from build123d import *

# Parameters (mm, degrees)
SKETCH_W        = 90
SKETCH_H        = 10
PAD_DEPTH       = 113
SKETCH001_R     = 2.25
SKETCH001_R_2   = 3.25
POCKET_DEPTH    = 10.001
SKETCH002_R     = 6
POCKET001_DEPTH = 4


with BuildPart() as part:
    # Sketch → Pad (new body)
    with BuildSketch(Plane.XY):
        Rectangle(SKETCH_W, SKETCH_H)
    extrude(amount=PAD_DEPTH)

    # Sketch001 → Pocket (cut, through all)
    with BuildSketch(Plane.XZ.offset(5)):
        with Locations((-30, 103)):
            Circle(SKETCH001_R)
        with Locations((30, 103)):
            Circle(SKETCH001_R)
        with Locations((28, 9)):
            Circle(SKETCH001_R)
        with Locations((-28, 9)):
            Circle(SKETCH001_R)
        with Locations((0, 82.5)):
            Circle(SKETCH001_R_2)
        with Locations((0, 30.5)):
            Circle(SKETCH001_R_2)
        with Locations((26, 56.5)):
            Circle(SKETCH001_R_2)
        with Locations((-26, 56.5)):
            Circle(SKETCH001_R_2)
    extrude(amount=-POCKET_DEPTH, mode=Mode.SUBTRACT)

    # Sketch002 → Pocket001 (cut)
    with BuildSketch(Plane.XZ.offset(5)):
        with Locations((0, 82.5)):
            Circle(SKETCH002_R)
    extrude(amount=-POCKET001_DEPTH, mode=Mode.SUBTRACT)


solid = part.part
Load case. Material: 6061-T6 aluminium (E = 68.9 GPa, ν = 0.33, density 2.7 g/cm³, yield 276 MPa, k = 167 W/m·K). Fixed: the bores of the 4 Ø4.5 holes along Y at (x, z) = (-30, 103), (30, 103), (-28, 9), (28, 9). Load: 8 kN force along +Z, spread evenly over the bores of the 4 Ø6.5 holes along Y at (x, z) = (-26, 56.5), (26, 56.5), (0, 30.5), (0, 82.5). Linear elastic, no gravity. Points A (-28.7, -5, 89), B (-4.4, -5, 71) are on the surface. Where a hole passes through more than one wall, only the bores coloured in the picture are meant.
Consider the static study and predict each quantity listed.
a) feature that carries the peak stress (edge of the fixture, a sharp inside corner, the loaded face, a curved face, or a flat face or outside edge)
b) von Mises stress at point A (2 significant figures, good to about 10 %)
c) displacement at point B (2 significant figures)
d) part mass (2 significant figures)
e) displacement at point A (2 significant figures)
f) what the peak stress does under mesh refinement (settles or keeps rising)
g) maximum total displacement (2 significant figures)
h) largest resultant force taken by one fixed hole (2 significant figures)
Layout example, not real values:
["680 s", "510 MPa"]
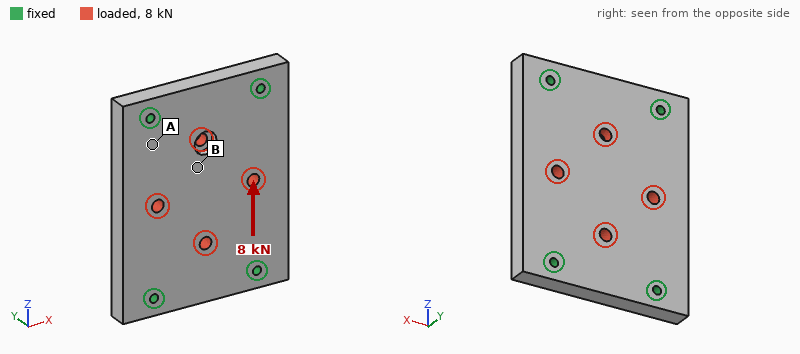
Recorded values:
["edge of the fixture", "7.5 MPa", "4.2 µm", "270 g", "1.8 µm", "keeps rising", "5.7 µm", "2.1 kN"]
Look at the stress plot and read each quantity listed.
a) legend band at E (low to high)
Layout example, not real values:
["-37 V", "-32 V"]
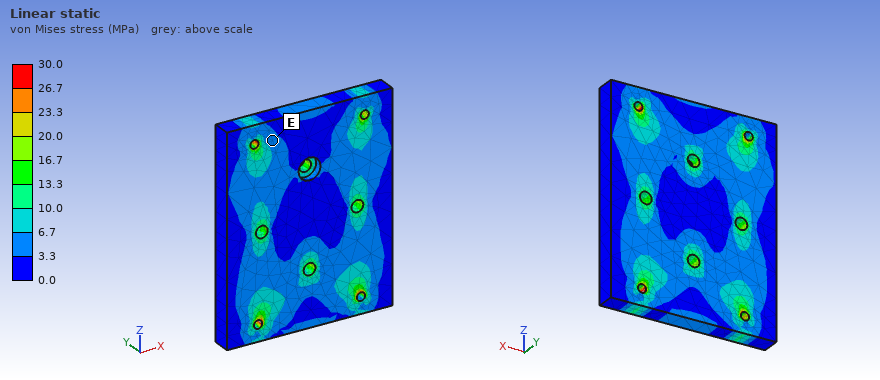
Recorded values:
["3.3 to 6.7 MPa"]
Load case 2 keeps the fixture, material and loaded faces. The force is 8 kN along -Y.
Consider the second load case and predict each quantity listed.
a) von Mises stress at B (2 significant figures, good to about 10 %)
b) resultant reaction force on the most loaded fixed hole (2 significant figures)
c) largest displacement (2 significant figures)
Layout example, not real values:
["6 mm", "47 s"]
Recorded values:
["26 MPa", "2.1 kN", "90 µm"]
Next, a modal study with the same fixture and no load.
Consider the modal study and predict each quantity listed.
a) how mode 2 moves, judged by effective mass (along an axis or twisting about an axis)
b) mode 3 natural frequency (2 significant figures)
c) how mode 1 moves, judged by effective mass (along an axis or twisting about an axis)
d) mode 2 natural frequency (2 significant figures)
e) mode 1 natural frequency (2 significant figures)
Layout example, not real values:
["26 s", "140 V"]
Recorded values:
["twisting about Z", "8800 Hz", "along Y", "5800 Hz", "4400 Hz"]
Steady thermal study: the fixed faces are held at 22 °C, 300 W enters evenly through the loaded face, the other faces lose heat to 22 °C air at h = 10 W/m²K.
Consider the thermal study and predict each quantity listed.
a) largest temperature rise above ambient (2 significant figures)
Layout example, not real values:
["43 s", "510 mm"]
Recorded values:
["52 K"]
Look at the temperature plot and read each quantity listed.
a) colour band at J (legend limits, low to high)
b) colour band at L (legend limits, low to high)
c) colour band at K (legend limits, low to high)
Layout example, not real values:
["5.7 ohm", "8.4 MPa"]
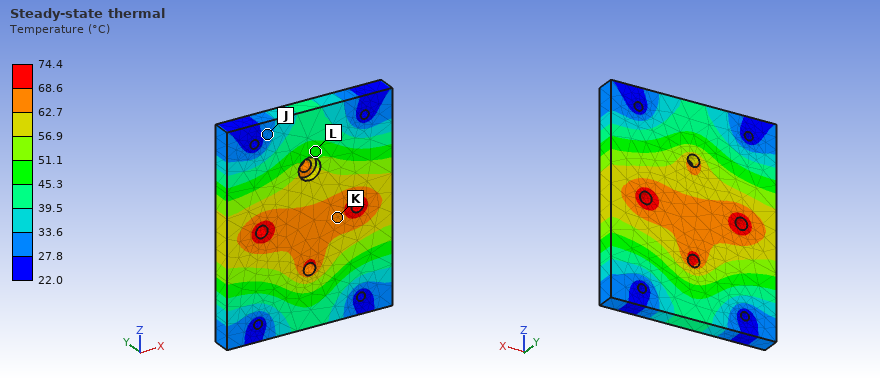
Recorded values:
["27.8 to 33.6 °C", "45.3 to 51.1 °C", "62.7 to 68.6 °C"]
